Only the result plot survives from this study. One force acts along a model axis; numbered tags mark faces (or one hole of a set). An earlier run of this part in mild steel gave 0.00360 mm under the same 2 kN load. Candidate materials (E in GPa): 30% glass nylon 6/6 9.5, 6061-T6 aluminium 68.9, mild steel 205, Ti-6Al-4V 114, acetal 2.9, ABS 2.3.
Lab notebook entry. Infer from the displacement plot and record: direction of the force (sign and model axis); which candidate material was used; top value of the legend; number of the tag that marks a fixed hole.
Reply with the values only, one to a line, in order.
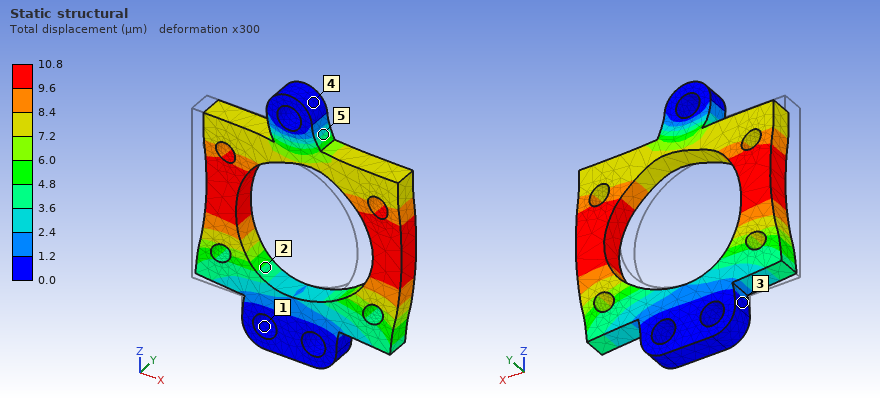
+X
6061-T6 aluminium
10.8 µm
1
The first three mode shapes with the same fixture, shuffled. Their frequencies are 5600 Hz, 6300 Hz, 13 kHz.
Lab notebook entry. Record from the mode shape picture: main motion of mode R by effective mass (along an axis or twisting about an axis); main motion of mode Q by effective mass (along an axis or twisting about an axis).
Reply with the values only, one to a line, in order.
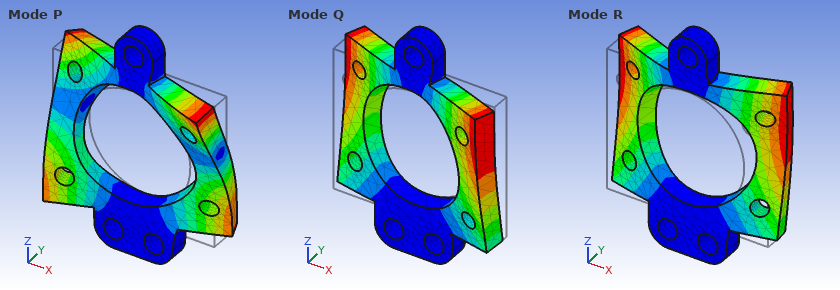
along Y
twisting about Z
